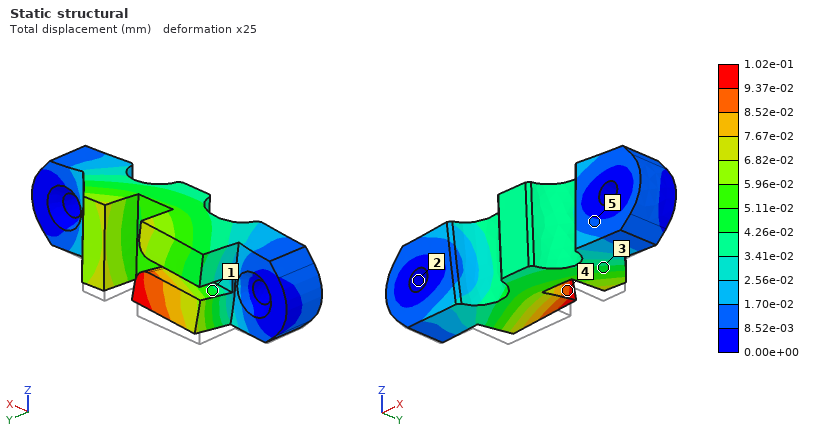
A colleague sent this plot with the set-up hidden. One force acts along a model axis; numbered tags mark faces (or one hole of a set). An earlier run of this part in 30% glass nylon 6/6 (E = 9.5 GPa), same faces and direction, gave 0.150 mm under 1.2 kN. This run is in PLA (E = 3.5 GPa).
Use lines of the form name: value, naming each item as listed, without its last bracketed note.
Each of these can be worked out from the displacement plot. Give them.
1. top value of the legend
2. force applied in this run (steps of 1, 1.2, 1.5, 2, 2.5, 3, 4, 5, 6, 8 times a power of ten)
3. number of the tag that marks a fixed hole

top value of the legend: 1.02e-01 mm
force applied in this run: 300 N
number of the tag that marks a fixed hole: 2
